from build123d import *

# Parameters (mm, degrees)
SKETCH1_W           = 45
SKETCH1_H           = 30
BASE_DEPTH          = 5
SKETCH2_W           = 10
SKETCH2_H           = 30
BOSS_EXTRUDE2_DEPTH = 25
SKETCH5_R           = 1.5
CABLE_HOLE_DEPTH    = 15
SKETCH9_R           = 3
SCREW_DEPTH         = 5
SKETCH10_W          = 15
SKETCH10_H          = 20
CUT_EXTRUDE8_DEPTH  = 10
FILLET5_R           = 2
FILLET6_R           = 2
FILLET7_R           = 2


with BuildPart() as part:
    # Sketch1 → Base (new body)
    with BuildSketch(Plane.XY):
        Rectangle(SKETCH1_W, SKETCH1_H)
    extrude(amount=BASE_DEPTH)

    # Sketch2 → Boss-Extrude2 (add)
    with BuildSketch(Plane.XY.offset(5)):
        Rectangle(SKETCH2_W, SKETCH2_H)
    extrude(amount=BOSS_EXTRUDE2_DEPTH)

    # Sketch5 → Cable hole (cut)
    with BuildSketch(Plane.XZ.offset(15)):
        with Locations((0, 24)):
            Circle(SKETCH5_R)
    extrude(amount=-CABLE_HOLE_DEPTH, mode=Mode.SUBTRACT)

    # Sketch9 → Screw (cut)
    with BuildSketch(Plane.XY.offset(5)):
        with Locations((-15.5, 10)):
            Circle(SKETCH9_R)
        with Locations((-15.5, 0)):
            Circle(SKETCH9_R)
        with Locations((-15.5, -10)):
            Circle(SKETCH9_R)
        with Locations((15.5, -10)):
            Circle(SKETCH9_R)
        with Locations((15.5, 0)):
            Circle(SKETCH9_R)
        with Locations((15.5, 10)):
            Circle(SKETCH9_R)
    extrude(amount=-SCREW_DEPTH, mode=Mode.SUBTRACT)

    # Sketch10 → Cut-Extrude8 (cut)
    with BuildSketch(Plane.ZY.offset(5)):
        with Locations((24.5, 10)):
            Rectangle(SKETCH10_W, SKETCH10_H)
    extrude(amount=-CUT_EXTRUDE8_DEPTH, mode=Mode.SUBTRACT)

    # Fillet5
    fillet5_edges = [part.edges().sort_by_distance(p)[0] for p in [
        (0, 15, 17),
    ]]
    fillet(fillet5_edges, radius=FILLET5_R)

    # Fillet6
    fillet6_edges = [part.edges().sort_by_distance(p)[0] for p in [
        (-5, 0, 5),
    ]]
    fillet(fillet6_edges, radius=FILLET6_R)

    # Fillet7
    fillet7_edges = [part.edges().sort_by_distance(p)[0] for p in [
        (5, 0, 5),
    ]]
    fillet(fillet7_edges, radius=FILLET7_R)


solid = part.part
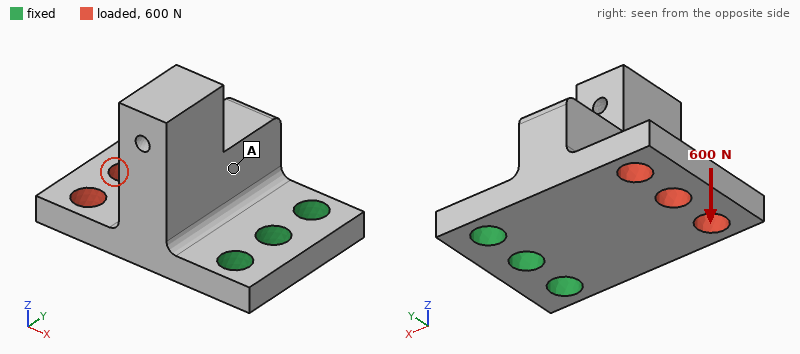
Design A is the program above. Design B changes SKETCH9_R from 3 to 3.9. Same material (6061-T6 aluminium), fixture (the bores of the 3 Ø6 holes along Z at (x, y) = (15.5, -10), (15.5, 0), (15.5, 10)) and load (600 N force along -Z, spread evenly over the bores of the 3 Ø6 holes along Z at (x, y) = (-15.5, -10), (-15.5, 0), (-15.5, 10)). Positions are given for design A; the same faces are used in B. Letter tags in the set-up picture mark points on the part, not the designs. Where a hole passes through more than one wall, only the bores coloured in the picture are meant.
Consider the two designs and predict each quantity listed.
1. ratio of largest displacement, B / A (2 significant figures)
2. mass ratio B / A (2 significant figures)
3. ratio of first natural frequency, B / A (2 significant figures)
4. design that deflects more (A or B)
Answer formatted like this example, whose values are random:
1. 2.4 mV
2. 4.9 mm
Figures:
1. 0.91
2. 0.95
3. 1.1
4. A
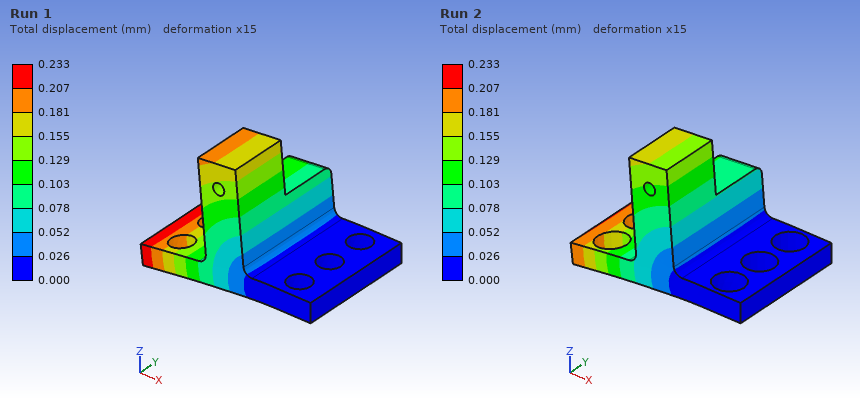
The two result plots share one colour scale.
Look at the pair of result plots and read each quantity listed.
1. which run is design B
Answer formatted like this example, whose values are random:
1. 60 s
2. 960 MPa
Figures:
1. Run 2
